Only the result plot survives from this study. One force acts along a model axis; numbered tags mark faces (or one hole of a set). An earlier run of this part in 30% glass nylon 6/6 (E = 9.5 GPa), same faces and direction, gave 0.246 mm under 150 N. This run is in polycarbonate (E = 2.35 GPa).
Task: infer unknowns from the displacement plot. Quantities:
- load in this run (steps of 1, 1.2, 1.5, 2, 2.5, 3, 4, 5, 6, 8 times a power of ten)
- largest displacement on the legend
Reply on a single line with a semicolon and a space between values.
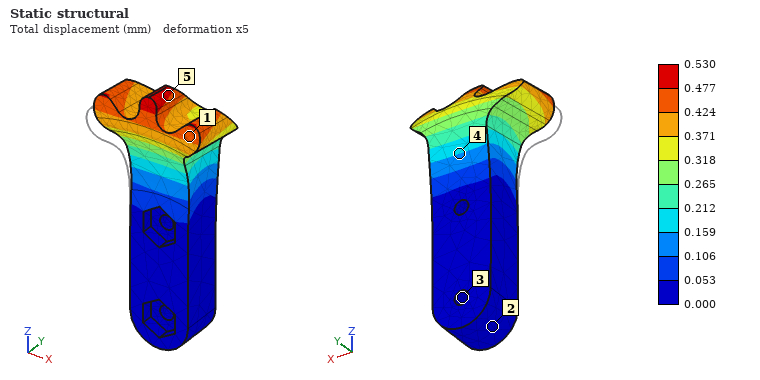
80 N; 0.530 mm
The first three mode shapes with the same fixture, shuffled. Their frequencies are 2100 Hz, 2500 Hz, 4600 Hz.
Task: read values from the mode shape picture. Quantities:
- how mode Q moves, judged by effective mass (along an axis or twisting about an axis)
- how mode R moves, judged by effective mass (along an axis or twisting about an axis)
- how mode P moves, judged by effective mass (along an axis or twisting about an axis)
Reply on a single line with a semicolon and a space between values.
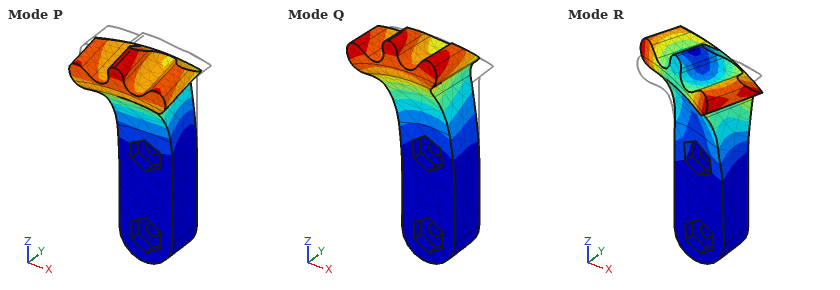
along X; twisting about Z; along Y
